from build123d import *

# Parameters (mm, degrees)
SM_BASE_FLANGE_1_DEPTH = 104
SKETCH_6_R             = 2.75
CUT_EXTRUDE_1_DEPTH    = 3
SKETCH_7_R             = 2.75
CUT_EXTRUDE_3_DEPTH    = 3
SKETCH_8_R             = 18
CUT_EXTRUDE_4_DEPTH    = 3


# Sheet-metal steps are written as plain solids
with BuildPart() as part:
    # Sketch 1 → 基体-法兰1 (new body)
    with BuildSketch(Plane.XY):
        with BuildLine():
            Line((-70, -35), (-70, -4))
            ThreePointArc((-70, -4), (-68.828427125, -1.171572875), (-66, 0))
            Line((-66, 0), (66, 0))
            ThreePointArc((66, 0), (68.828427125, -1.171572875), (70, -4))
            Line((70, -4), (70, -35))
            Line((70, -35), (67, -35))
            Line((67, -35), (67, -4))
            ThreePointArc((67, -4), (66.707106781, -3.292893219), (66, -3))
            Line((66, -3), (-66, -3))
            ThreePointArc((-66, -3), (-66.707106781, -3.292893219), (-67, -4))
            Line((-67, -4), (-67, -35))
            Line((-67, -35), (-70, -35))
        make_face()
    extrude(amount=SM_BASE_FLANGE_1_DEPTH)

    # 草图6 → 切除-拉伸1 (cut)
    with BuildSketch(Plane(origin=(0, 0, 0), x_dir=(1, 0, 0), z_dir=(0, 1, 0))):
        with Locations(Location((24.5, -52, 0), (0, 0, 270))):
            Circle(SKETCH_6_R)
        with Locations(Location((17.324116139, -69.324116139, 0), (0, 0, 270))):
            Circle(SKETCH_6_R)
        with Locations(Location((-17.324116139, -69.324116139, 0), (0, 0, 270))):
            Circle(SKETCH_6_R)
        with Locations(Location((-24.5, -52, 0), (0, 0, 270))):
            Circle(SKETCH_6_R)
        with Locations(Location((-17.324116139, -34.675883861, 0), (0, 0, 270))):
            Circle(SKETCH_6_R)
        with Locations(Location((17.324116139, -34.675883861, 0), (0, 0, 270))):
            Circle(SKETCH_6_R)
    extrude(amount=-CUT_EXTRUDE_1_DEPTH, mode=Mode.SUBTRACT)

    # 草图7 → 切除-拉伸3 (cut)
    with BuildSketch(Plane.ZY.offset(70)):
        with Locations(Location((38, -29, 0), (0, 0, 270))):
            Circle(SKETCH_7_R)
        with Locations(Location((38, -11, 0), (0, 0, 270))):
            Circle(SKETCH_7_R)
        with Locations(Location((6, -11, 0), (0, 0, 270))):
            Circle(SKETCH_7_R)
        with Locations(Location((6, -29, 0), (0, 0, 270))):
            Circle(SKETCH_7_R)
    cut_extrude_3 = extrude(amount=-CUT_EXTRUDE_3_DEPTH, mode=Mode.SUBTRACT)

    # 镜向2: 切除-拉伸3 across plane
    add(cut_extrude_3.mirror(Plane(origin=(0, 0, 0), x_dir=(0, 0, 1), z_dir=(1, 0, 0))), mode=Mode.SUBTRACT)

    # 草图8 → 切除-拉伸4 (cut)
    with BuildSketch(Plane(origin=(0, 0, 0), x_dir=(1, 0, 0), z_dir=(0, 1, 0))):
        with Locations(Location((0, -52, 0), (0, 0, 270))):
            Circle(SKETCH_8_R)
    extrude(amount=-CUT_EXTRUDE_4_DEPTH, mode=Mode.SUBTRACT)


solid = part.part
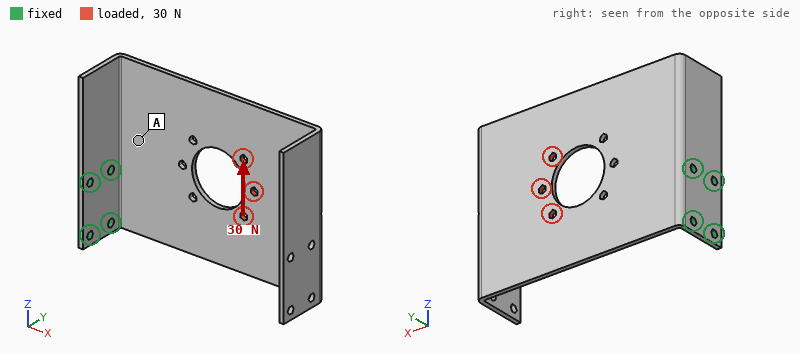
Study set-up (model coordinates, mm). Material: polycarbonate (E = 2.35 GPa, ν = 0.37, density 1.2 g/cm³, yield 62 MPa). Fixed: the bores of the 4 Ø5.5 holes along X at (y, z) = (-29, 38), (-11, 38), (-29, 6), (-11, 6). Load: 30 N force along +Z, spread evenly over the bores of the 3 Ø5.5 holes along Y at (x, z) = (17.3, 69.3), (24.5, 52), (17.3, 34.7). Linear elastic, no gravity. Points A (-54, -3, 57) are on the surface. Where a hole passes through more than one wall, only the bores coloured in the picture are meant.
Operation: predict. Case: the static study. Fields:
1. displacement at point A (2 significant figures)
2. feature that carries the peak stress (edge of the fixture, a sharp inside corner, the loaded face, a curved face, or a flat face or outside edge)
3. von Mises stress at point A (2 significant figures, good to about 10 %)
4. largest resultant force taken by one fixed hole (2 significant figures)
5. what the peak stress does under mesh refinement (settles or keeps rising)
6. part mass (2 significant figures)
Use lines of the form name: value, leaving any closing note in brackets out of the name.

displacement at point A: 0.25 mm
feature that carries the peak stress: edge of the fixture
von Mises stress at point A: 0.90 MPa
largest resultant force taken by one fixed hole: 82 N
what the peak stress does under mesh refinement: keeps rising
part mass: 71 g
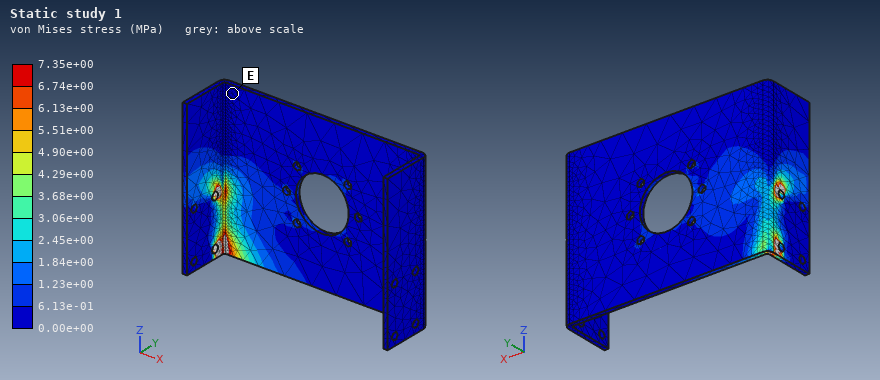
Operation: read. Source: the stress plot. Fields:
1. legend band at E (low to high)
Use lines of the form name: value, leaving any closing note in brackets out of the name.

legend band at E: 0.00e+00 to 6.13e-01 MPa
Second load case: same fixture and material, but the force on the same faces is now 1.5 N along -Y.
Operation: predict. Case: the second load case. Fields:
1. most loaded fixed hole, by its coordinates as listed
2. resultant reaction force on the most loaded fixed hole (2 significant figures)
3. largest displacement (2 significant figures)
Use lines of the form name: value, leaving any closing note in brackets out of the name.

most loaded fixed hole, by its coordinates as listed: (-11, 38)
resultant reaction force on the most loaded fixed hole: 3.9 N
largest displacement: 1.8 mm
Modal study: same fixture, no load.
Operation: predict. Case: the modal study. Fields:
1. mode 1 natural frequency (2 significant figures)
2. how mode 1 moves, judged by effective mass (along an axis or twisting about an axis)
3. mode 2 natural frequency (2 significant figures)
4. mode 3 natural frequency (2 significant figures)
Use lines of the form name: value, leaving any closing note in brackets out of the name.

mode 1 natural frequency: 22 Hz
how mode 1 moves, judged by effective mass: along Y
mode 2 natural frequency: 70 Hz
mode 3 natural frequency: 130 Hz
